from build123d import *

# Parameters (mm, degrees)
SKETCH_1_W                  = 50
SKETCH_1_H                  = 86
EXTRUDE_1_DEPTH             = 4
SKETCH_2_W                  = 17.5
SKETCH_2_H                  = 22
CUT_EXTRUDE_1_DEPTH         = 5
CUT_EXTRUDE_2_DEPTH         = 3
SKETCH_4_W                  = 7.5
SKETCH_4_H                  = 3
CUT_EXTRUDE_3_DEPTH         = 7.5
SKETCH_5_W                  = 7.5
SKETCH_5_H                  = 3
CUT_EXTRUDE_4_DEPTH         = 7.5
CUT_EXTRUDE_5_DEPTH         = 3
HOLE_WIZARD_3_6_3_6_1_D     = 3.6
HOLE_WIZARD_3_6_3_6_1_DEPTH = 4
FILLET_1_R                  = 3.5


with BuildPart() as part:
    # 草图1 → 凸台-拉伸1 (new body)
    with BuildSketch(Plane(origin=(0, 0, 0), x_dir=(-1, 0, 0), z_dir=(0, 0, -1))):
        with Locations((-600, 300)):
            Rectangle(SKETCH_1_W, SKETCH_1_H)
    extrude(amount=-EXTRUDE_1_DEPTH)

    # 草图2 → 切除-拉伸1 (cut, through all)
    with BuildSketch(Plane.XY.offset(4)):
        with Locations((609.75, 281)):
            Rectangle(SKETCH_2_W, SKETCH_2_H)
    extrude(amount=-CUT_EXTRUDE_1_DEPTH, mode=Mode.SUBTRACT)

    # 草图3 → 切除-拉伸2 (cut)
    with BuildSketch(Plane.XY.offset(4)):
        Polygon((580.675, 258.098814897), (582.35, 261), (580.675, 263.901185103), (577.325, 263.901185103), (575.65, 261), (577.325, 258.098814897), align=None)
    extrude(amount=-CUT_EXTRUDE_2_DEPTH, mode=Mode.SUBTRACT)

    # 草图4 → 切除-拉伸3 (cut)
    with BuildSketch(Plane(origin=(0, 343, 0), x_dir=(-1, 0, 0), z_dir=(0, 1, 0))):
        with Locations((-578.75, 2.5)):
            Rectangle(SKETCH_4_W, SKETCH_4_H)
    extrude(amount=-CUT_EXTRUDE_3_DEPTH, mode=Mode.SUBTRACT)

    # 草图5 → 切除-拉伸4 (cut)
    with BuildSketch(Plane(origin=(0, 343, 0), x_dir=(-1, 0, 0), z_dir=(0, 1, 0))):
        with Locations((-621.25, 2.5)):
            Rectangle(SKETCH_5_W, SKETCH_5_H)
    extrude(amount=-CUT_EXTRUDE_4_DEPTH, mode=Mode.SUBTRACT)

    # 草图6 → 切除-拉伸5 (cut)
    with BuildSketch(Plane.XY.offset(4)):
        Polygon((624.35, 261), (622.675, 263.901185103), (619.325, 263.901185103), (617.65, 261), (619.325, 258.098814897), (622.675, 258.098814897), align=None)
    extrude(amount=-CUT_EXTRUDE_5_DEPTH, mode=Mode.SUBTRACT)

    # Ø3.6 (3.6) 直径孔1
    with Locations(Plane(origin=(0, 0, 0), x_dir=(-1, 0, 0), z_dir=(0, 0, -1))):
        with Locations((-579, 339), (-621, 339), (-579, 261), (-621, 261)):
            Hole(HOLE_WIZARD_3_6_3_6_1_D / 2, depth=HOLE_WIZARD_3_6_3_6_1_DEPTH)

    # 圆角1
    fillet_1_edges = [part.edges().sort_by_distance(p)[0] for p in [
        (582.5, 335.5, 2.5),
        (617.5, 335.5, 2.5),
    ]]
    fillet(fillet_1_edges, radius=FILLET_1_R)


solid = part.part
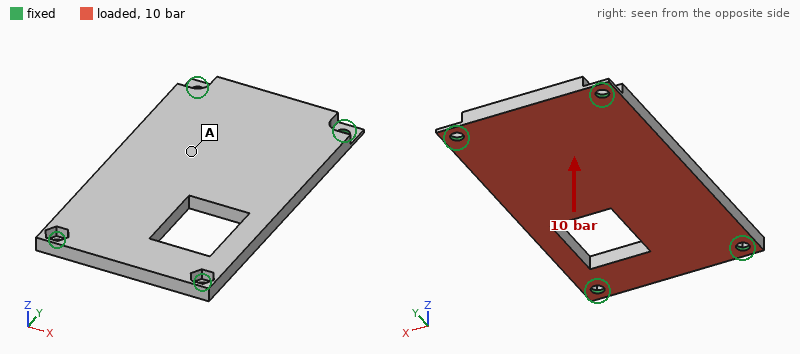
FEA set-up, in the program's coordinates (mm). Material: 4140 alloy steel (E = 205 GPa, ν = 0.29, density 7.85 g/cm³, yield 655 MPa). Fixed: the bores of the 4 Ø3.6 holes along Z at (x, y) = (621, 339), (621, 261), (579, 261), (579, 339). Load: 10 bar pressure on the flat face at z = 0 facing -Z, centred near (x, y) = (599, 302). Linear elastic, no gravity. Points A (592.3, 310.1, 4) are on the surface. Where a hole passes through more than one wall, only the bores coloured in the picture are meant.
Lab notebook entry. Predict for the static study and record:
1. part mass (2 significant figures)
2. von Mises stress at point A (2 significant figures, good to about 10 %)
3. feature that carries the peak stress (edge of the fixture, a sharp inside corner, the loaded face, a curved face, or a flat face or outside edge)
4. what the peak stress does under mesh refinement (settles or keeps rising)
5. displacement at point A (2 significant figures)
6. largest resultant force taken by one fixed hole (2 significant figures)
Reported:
120 g
140 MPa
edge of the fixture
keeps rising
0.20 mm
3.2 kN
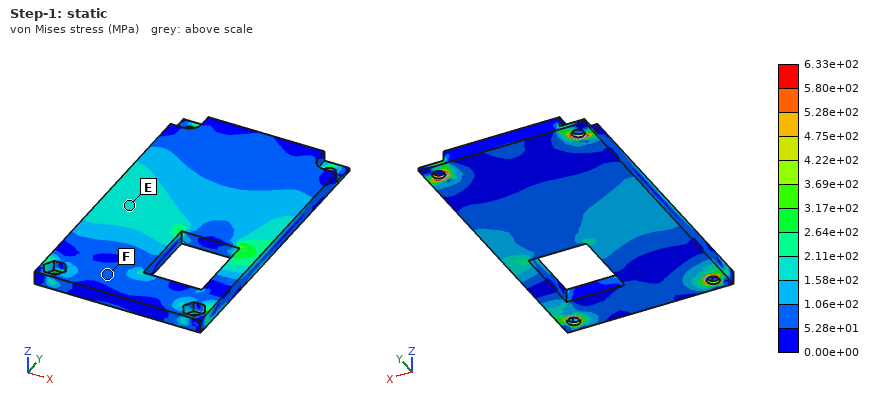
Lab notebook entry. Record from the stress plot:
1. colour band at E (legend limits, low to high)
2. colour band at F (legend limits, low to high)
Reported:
1.58e+02 to 2.11e+02 MPa
5.28e+01 to 1.06e+02 MPa
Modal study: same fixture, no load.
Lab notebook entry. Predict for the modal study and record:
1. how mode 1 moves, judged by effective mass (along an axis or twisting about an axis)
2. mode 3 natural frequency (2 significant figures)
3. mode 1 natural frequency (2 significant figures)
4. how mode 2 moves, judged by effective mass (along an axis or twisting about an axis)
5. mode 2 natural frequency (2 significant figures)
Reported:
along Z
6000 Hz
2100 Hz
twisting about Y
3900 Hz
